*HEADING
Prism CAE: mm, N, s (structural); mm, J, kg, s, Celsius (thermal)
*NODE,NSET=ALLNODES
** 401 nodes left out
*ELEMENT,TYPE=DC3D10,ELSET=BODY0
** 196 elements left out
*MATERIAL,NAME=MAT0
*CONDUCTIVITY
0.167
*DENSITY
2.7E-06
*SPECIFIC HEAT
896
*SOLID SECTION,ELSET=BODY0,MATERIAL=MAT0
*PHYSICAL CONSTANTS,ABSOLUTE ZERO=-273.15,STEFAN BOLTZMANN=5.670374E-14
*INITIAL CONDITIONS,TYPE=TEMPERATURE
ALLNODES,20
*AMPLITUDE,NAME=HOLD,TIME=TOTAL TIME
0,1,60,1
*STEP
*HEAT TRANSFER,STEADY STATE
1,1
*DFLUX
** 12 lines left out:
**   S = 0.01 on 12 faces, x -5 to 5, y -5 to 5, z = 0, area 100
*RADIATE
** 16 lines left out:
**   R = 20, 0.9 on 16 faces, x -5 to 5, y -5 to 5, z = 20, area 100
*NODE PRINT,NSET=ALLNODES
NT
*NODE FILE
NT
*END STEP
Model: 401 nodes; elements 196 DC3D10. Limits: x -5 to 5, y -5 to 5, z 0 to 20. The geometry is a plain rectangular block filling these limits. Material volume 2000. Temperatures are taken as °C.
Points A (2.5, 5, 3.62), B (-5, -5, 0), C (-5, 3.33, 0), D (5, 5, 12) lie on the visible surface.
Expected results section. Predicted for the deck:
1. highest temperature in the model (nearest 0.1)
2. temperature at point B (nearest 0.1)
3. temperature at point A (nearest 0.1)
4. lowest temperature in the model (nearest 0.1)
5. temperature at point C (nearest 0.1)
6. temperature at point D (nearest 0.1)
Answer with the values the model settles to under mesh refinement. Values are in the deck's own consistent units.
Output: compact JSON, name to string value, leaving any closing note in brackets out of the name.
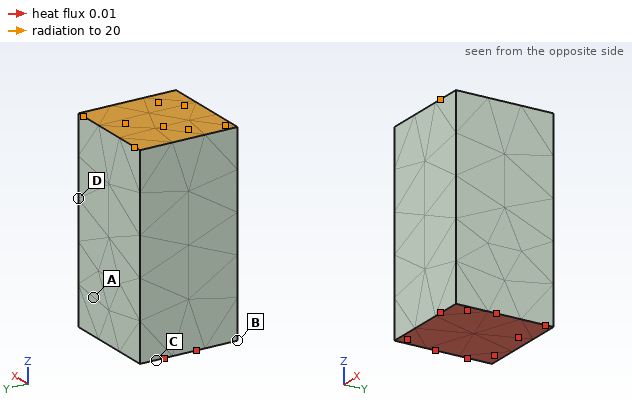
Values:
{"highest temperature in the model": "399.6 °C", "temperature at point B": "399.6 °C", "temperature at point A": "399.3 °C", "lowest temperature in the model": "398.4 °C", "temperature at point C": "399.6 °C", "temperature at point D": "398.8 °C"}
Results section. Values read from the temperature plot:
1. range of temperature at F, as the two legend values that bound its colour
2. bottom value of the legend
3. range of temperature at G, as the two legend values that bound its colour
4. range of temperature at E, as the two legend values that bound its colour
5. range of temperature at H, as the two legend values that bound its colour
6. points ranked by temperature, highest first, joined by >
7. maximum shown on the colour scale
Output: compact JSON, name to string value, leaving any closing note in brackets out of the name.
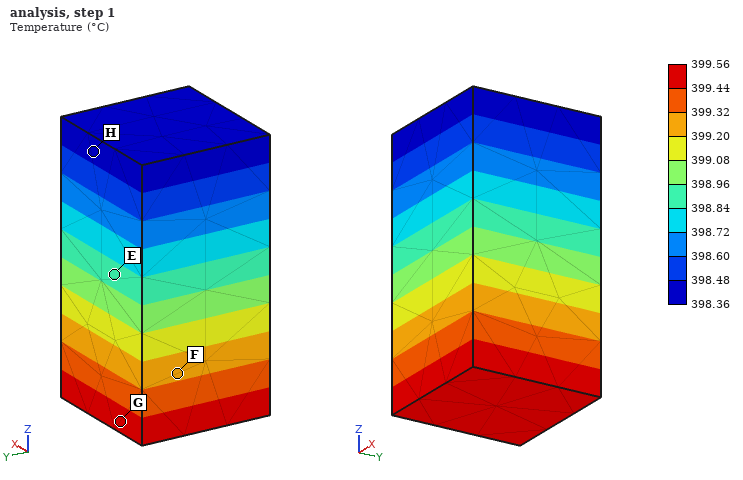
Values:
{"range of temperature at F, as the two legend values that bound its colour": "399.20 to 399.32 °C", "bottom value of the legend": "398.36 °C", "range of temperature at G, as the two legend values that bound its colour": "399.44 to 399.56 °C", "range of temperature at E, as the two legend values that bound its colour": "398.84 to 398.96 °C", "range of temperature at H, as the two legend values that bound its colour": "398.36 to 398.48 °C", "points ranked by temperature, highest first, joined by >": "G > F > E > H", "maximum shown on the colour scale": "399.56 °C"}
